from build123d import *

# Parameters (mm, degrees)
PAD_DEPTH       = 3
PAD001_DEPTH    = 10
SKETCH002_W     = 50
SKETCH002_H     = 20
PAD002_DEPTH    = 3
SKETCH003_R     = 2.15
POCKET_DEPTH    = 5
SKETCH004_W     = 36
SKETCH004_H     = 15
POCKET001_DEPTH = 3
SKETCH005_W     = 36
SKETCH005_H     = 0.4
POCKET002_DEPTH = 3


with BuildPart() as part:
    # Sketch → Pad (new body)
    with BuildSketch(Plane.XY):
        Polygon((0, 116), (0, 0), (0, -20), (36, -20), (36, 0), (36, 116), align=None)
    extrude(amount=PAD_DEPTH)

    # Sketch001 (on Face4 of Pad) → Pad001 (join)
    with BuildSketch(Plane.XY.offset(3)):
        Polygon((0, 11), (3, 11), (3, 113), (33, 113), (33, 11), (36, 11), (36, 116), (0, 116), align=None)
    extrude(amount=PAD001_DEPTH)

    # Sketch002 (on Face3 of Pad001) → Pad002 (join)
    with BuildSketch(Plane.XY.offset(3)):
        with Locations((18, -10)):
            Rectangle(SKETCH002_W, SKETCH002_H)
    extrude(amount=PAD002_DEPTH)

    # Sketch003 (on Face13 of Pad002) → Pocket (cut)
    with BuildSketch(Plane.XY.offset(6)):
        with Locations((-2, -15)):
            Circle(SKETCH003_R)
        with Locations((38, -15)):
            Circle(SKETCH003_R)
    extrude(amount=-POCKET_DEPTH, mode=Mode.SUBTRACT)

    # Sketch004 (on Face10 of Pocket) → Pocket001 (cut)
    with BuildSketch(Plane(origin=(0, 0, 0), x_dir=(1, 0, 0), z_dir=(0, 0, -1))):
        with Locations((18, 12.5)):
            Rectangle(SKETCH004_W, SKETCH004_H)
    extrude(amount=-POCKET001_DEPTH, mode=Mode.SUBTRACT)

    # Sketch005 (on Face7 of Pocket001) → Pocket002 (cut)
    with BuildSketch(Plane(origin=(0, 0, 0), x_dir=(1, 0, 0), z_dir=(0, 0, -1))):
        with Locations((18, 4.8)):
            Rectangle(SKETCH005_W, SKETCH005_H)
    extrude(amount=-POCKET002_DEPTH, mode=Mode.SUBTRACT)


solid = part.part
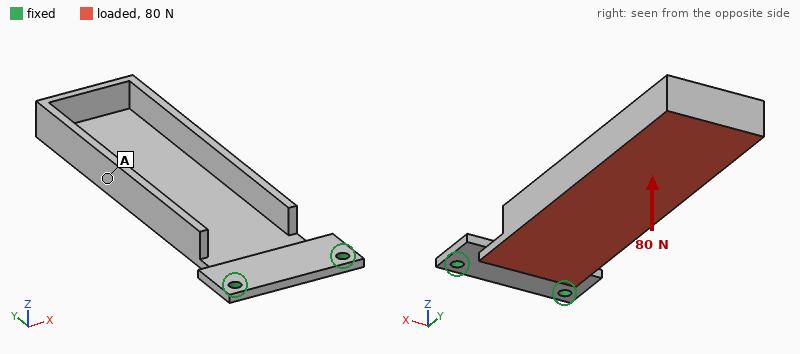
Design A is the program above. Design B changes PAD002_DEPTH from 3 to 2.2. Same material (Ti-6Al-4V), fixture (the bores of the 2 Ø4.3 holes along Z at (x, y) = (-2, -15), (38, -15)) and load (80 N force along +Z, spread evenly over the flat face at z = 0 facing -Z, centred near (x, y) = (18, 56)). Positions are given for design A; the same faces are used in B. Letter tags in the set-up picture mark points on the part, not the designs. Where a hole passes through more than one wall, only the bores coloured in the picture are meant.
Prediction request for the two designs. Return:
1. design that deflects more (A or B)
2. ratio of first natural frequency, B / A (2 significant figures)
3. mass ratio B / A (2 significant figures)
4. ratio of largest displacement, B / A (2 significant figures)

B
0.78
0.97
1.6
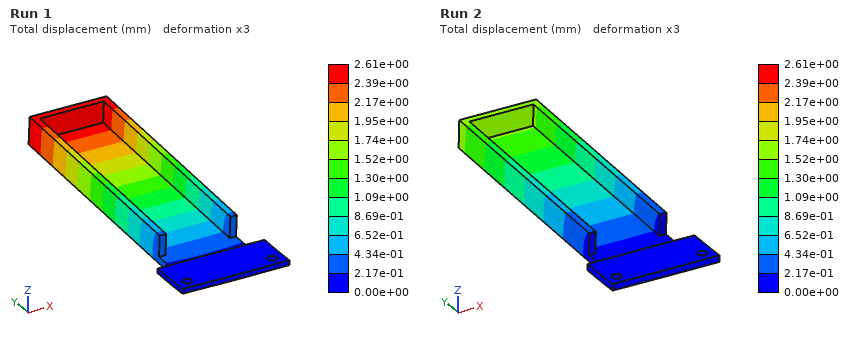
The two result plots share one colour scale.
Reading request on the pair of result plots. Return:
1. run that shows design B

Run 1
